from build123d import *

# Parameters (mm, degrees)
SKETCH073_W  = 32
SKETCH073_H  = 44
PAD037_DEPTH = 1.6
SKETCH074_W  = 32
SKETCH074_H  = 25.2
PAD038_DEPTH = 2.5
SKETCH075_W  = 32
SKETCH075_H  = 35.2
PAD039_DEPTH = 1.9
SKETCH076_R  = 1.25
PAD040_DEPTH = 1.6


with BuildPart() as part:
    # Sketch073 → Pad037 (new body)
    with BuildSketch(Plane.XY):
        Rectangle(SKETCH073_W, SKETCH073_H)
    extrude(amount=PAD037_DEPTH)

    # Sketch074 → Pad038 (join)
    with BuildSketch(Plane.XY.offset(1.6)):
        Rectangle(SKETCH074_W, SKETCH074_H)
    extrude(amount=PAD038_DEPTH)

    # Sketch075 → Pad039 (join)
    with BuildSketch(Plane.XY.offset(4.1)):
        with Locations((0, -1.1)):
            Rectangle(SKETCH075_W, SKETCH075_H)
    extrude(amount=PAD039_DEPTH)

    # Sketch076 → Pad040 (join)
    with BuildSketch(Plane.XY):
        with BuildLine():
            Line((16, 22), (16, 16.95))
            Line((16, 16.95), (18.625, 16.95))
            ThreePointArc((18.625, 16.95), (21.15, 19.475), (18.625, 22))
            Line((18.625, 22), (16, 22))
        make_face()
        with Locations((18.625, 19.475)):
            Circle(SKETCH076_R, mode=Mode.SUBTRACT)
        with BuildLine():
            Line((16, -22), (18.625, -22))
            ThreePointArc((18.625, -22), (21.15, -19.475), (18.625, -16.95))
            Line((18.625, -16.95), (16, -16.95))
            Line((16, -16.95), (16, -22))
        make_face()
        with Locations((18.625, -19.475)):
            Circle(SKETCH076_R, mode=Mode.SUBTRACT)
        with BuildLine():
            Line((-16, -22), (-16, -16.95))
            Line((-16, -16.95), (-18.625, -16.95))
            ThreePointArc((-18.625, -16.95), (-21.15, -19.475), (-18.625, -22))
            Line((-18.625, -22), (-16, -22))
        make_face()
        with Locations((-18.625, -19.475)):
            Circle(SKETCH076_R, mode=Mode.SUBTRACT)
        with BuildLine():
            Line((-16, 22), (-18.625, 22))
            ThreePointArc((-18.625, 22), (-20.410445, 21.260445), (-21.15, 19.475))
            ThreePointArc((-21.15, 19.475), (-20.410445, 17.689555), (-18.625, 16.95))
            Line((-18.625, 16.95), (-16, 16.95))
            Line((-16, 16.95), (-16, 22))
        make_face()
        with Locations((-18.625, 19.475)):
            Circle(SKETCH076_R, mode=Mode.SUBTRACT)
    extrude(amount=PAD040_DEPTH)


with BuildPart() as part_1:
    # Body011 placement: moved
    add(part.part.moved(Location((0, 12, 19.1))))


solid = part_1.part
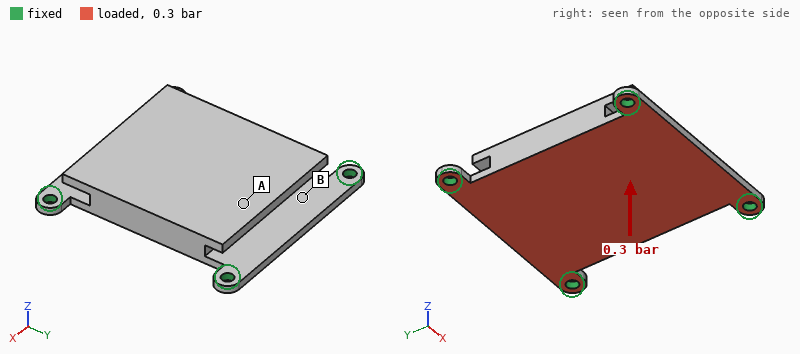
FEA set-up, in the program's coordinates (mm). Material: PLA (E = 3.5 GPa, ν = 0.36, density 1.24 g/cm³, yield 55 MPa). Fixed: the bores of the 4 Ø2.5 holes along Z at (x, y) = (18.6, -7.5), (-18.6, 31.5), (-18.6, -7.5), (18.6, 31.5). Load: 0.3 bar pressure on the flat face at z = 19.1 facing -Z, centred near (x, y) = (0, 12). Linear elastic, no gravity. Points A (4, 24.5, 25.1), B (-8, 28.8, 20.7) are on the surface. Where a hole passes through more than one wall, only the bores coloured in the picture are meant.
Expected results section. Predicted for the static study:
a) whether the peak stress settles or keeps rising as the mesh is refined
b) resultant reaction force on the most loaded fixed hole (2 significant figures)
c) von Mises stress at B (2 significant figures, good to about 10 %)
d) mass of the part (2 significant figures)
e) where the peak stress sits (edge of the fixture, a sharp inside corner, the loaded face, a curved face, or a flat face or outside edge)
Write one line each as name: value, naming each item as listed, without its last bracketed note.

whether the peak stress settles or keeps rising as the mesh is refined: keeps rising
resultant reaction force on the most loaded fixed hole: 12 N
von Mises stress at B: 3.2 MPa
mass of the part: 8.1 g
where the peak stress sits: edge of the fixture
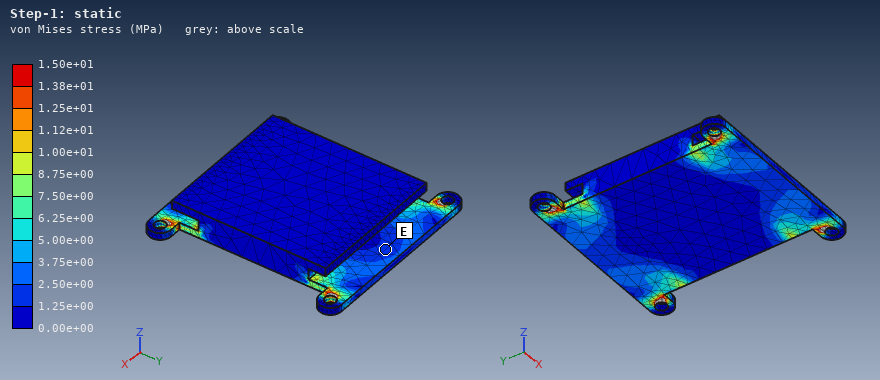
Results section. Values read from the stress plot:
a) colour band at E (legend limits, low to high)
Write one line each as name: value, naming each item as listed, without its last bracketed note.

colour band at E: 1.25e+00 to 2.50e+00 MPa
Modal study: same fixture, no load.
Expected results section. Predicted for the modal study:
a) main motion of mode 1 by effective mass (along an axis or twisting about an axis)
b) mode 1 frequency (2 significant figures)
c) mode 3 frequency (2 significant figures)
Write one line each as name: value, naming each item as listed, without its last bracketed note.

main motion of mode 1 by effective mass: along Z
mode 1 frequency: 1200 Hz
mode 3 frequency: 2100 Hz
